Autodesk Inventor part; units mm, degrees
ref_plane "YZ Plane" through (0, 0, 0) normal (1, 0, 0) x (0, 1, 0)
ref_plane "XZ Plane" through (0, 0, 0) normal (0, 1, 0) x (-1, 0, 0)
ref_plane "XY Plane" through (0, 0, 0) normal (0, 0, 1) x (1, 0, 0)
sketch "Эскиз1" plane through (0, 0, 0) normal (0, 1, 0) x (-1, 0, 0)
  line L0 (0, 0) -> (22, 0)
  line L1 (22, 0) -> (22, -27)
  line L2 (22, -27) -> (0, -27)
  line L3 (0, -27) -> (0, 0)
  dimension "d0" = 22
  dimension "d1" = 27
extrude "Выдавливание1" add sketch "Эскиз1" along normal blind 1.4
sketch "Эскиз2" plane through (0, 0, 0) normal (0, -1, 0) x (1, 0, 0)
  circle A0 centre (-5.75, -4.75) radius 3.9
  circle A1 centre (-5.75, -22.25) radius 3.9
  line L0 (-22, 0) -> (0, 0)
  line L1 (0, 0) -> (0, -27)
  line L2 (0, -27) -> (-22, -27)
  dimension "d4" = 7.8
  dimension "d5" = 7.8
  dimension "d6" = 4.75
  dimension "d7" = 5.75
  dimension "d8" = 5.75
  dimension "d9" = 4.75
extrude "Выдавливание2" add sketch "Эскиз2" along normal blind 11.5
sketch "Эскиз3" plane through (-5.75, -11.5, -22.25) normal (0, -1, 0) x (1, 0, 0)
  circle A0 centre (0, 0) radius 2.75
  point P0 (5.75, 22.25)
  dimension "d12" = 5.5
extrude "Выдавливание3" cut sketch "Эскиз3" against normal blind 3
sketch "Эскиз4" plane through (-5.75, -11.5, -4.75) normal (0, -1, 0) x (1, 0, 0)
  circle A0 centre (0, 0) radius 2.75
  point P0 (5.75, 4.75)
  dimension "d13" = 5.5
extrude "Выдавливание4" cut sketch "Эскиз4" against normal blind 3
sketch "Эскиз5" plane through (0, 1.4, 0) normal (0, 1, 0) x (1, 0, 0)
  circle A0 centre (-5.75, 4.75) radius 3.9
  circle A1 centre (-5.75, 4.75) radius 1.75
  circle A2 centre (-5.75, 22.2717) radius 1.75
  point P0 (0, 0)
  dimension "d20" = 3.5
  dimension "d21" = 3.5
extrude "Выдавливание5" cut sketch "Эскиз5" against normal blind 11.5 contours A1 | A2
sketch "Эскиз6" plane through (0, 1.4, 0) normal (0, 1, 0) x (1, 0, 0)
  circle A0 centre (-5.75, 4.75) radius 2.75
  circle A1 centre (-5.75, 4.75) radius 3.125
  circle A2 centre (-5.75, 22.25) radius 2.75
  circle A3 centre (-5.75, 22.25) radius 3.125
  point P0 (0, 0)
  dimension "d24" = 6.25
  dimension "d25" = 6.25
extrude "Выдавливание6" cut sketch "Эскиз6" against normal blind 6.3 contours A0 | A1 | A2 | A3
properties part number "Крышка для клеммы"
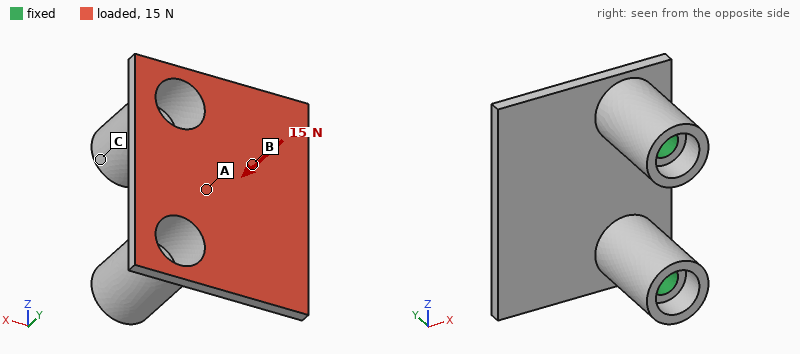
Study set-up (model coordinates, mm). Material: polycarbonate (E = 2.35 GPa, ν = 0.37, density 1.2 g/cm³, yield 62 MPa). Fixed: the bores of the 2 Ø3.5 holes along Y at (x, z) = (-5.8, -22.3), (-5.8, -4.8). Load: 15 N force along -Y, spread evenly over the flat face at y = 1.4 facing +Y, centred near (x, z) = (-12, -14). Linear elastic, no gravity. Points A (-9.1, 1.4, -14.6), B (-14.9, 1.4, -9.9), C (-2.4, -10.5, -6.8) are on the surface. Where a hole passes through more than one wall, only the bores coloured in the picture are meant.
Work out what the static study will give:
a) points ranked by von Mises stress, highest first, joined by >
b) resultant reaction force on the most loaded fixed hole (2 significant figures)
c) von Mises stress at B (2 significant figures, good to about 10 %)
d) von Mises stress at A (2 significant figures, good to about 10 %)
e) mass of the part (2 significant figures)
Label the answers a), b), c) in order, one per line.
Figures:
a) A > B > C
b) 7.6 N
c) 2.2 MPa
d) 4.7 MPa
e) 1.6 g
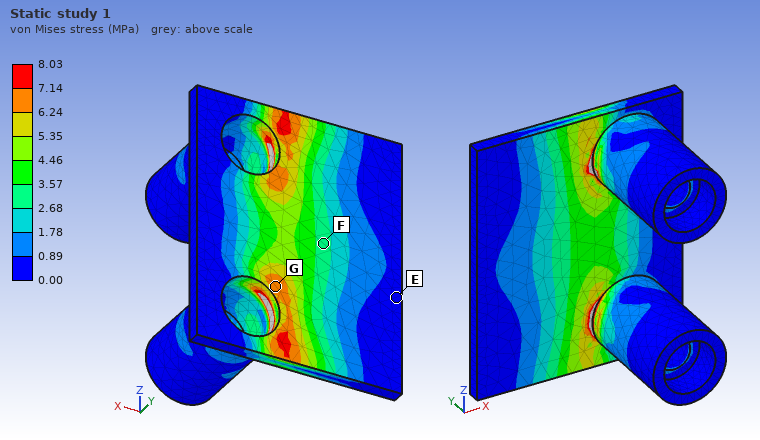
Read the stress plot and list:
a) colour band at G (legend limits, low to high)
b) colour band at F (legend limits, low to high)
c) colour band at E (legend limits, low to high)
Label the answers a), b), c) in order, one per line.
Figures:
a) 6.24 to 7.14 MPa
b) 2.68 to 3.57 MPa
c) 0.00 to 0.89 MPa
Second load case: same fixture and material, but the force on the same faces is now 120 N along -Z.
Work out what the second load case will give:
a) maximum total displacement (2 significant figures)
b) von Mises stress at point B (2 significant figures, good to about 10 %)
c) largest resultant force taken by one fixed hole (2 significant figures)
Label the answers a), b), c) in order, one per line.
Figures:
a) 0.23 mm
b) 4.5 MPa
c) 67 N
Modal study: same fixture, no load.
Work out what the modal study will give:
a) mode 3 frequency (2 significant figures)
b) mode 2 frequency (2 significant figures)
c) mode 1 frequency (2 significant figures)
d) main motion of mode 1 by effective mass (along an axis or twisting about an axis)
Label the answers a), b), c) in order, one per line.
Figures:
a) 4400 Hz
b) 2300 Hz
c) 1400 Hz
d) along Y
